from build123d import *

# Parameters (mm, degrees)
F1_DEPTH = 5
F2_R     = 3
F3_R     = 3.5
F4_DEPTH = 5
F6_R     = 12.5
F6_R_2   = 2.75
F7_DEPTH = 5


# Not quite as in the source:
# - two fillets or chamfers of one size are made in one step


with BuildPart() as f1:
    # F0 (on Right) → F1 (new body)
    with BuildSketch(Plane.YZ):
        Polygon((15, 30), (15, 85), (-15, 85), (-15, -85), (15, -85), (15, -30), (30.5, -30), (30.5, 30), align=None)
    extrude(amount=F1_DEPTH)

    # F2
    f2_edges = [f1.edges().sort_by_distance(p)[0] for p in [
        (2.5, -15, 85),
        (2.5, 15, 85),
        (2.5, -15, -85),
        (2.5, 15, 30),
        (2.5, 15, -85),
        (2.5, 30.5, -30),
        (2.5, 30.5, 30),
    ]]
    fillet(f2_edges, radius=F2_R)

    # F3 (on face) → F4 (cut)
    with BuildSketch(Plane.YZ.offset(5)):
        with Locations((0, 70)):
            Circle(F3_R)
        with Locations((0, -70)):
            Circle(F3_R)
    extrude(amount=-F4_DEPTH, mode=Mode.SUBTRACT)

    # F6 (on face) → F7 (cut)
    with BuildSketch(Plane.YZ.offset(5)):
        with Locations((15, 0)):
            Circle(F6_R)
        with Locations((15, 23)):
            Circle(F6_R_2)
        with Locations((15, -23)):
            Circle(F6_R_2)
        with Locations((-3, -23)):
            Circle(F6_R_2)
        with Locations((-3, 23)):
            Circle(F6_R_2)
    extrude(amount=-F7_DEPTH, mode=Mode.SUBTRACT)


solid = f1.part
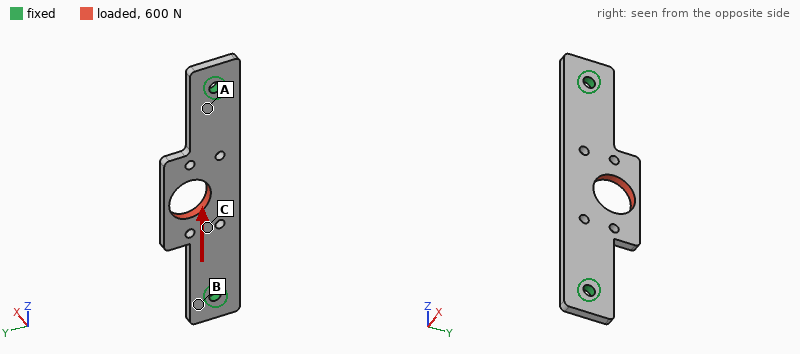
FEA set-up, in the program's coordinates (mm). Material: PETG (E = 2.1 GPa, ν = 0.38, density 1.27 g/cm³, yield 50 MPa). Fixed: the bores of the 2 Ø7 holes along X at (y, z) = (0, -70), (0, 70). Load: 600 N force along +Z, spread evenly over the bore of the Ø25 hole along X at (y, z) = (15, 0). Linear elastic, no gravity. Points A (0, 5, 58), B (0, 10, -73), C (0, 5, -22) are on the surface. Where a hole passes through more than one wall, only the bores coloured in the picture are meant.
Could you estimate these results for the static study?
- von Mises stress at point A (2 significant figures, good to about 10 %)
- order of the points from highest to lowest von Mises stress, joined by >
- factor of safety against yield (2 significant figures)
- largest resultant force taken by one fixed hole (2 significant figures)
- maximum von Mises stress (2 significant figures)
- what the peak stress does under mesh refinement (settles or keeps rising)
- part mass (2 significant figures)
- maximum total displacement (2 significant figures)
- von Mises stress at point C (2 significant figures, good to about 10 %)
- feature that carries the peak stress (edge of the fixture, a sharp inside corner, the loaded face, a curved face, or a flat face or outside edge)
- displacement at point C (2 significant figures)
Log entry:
3.2 MPa
A > C > B
3.0
310 N
17 MPa
settles
34 g
0.18 mm
1.7 MPa
a curved face
0.058 mm
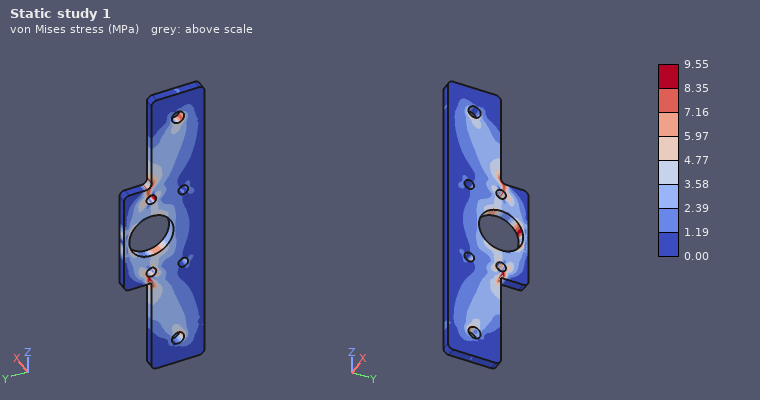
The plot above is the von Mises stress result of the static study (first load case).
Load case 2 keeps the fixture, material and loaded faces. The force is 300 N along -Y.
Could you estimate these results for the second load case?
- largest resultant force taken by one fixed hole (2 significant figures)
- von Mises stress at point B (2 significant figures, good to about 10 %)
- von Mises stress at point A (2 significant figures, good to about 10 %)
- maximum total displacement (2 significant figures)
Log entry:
150 N
1.8 MPa
2.4 MPa
0.36 mm
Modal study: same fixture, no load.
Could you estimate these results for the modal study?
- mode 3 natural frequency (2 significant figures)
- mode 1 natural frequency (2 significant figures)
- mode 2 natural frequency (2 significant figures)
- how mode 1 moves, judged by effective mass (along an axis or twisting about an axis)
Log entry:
820 Hz
310 Hz
570 Hz
along X
